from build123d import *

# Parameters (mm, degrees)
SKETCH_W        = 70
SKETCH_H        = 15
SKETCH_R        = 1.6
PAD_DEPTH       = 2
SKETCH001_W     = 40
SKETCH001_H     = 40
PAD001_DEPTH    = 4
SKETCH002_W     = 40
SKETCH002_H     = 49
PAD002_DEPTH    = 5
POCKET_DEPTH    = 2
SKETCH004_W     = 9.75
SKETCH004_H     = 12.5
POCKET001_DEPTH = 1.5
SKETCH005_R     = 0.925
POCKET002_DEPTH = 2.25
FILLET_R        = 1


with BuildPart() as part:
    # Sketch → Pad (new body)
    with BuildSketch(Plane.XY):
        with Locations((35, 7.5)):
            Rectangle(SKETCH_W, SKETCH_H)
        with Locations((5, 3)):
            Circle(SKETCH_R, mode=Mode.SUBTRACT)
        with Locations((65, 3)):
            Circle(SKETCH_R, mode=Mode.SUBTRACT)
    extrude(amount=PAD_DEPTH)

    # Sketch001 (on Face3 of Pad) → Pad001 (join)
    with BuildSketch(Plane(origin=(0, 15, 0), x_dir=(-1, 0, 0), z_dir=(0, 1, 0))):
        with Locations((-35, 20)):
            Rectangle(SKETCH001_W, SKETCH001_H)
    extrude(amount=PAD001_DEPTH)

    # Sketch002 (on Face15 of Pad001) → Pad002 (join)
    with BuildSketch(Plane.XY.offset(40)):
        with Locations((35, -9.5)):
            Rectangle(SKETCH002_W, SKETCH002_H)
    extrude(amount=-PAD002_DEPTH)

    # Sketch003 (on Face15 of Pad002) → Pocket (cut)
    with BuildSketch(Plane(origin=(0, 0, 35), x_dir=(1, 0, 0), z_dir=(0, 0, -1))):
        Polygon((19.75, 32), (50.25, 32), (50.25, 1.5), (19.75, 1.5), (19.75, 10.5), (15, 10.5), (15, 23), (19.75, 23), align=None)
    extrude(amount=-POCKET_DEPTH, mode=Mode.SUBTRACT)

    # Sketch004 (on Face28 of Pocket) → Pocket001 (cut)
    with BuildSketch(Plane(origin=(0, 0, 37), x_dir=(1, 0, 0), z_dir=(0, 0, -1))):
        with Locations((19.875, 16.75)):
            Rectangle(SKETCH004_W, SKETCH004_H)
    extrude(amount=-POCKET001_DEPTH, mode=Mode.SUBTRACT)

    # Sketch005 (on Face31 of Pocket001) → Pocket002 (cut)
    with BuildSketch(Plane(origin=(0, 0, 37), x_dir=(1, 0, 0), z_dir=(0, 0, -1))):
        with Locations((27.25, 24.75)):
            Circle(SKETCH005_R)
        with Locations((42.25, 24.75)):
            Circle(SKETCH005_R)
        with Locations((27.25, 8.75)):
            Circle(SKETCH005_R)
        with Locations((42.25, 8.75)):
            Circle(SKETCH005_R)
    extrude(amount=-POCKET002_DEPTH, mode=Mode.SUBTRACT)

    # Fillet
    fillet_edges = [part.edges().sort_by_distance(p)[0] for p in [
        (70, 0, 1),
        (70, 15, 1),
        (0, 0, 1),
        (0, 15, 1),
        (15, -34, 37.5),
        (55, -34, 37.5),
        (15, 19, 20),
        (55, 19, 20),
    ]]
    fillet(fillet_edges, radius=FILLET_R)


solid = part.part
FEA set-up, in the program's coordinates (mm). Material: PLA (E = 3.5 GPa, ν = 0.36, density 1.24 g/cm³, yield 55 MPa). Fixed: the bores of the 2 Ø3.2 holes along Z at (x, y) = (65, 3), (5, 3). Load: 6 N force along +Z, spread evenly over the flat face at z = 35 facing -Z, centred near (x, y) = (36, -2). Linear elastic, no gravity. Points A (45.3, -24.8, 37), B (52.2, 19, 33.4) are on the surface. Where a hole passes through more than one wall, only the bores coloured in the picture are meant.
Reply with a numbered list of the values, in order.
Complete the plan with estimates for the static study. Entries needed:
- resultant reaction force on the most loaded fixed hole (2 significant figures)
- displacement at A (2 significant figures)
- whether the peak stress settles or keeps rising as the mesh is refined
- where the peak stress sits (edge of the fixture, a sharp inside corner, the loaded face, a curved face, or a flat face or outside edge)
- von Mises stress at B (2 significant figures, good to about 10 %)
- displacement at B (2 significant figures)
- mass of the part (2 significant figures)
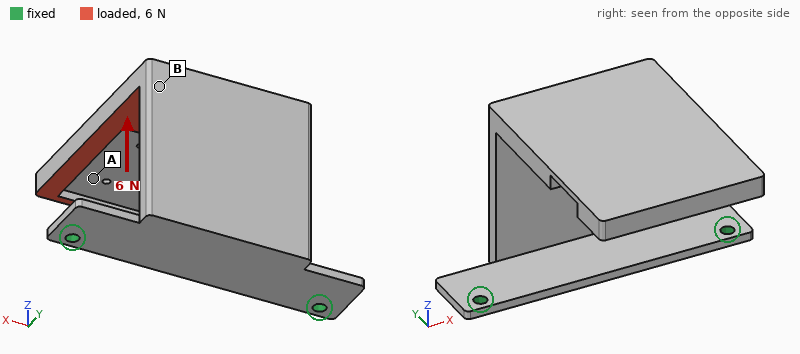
1. 3.1 N
2. 0.96 mm
3. keeps rising
4. a sharp inside corner
5. 0.94 MPa
6. 0.52 mm
7. 20 g
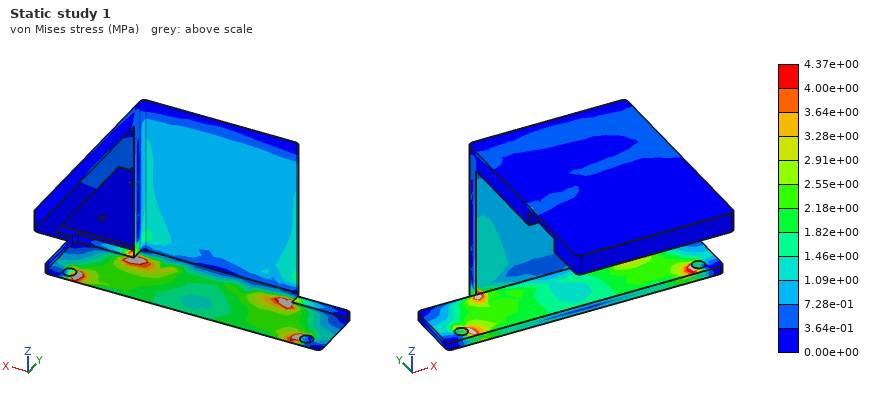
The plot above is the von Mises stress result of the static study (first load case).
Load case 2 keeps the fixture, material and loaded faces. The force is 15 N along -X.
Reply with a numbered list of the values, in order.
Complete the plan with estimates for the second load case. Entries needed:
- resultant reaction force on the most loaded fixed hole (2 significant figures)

1. 13 N
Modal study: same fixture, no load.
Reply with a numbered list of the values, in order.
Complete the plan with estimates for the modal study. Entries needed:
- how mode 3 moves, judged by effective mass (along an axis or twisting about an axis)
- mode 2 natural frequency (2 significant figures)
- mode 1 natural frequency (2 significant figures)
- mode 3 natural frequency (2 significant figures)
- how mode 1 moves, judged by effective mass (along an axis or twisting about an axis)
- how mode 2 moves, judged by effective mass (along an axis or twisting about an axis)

1. along Z
2. 210 Hz
3. 72 Hz
4. 300 Hz
5. along Y
6. along X
